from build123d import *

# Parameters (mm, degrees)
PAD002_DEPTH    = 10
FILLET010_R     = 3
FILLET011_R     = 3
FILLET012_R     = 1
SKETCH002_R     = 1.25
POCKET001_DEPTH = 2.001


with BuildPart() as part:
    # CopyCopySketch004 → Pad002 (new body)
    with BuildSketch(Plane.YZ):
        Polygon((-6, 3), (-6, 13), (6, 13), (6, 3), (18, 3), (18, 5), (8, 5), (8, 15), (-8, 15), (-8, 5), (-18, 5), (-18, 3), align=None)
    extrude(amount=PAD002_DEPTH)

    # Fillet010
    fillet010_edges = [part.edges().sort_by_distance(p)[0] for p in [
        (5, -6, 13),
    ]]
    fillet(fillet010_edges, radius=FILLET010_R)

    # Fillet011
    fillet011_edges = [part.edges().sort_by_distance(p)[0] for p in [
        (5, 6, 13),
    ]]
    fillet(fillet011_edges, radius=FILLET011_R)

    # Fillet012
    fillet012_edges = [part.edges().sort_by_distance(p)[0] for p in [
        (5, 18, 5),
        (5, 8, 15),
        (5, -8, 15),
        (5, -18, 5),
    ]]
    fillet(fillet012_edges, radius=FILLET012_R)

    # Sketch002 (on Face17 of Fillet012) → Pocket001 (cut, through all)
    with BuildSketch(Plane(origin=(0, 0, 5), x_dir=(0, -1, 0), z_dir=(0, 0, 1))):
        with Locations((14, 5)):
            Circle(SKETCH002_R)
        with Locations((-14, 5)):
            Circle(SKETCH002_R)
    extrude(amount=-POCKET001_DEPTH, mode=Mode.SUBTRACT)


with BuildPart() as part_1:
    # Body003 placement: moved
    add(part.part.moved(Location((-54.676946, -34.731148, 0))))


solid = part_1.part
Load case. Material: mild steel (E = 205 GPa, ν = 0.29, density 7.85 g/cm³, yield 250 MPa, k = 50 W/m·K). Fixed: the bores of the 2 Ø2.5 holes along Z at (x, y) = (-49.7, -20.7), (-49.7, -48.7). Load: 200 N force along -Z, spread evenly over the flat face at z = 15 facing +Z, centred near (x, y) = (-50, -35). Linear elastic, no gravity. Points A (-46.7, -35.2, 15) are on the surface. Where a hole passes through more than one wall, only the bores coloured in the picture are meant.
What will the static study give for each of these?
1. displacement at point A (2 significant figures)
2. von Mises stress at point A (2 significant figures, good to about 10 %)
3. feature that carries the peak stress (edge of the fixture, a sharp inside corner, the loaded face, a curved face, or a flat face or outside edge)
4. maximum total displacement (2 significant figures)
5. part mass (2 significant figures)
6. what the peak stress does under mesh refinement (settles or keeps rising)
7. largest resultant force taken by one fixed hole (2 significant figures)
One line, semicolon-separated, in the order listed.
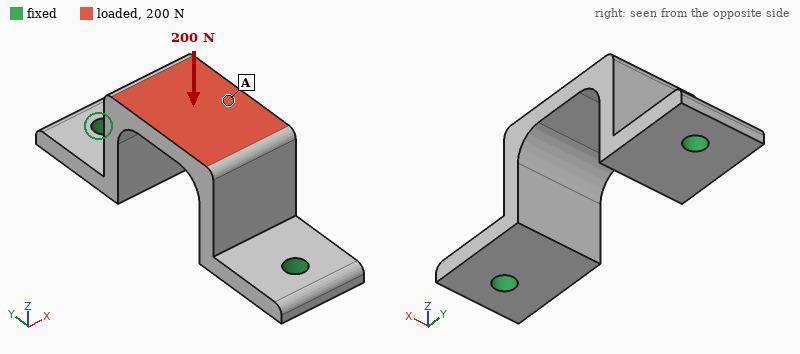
3.9 µm; 13 MPa; edge of the fixture; 4.0 µm; 8.9 g; keeps rising; 110 N
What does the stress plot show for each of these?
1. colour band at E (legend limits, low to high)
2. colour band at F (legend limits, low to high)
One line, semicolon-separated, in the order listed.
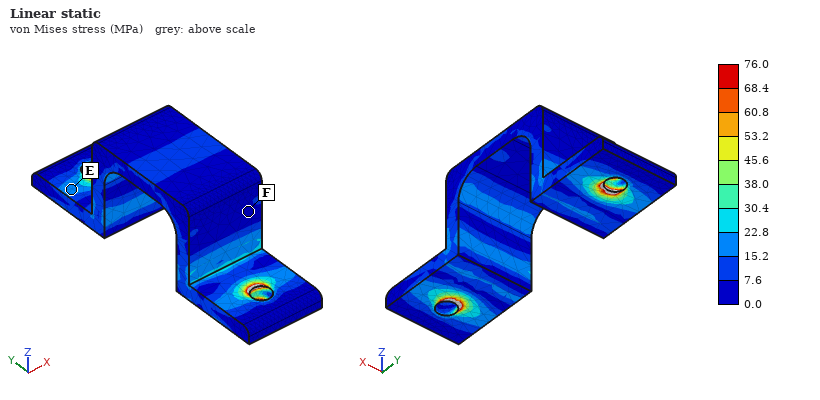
15.2 to 22.8 MPa; 0.0 to 7.6 MPa
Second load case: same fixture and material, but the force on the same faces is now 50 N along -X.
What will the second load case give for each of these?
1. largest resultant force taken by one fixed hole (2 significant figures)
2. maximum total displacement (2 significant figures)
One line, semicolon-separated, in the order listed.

25 N; 9.7 µm
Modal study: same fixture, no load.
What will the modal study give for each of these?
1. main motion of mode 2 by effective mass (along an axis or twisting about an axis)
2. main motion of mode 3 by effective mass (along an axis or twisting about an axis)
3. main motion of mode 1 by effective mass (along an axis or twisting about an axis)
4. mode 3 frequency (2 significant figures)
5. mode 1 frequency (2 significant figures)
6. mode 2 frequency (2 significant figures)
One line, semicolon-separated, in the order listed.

along Y; along Z; along X; 15 kHz; 6600 Hz; 13 kHz
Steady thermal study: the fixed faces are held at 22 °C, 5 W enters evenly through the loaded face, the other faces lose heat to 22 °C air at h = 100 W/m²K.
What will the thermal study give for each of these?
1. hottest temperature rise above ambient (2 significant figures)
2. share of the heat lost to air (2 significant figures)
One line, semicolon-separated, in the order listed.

33 K; 34 %
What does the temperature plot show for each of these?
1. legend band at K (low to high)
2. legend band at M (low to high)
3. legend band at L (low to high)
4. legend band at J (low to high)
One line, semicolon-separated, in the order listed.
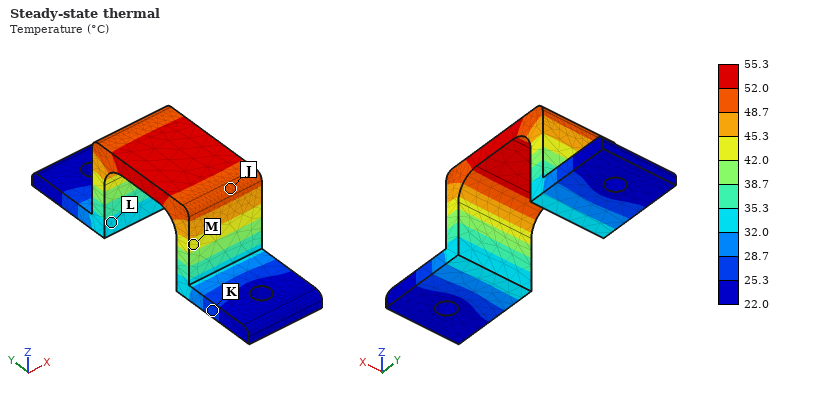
25.3 to 28.7 °C; 42.0 to 45.3 °C; 32.0 to 35.3 °C; 48.7 to 52.0 °C
